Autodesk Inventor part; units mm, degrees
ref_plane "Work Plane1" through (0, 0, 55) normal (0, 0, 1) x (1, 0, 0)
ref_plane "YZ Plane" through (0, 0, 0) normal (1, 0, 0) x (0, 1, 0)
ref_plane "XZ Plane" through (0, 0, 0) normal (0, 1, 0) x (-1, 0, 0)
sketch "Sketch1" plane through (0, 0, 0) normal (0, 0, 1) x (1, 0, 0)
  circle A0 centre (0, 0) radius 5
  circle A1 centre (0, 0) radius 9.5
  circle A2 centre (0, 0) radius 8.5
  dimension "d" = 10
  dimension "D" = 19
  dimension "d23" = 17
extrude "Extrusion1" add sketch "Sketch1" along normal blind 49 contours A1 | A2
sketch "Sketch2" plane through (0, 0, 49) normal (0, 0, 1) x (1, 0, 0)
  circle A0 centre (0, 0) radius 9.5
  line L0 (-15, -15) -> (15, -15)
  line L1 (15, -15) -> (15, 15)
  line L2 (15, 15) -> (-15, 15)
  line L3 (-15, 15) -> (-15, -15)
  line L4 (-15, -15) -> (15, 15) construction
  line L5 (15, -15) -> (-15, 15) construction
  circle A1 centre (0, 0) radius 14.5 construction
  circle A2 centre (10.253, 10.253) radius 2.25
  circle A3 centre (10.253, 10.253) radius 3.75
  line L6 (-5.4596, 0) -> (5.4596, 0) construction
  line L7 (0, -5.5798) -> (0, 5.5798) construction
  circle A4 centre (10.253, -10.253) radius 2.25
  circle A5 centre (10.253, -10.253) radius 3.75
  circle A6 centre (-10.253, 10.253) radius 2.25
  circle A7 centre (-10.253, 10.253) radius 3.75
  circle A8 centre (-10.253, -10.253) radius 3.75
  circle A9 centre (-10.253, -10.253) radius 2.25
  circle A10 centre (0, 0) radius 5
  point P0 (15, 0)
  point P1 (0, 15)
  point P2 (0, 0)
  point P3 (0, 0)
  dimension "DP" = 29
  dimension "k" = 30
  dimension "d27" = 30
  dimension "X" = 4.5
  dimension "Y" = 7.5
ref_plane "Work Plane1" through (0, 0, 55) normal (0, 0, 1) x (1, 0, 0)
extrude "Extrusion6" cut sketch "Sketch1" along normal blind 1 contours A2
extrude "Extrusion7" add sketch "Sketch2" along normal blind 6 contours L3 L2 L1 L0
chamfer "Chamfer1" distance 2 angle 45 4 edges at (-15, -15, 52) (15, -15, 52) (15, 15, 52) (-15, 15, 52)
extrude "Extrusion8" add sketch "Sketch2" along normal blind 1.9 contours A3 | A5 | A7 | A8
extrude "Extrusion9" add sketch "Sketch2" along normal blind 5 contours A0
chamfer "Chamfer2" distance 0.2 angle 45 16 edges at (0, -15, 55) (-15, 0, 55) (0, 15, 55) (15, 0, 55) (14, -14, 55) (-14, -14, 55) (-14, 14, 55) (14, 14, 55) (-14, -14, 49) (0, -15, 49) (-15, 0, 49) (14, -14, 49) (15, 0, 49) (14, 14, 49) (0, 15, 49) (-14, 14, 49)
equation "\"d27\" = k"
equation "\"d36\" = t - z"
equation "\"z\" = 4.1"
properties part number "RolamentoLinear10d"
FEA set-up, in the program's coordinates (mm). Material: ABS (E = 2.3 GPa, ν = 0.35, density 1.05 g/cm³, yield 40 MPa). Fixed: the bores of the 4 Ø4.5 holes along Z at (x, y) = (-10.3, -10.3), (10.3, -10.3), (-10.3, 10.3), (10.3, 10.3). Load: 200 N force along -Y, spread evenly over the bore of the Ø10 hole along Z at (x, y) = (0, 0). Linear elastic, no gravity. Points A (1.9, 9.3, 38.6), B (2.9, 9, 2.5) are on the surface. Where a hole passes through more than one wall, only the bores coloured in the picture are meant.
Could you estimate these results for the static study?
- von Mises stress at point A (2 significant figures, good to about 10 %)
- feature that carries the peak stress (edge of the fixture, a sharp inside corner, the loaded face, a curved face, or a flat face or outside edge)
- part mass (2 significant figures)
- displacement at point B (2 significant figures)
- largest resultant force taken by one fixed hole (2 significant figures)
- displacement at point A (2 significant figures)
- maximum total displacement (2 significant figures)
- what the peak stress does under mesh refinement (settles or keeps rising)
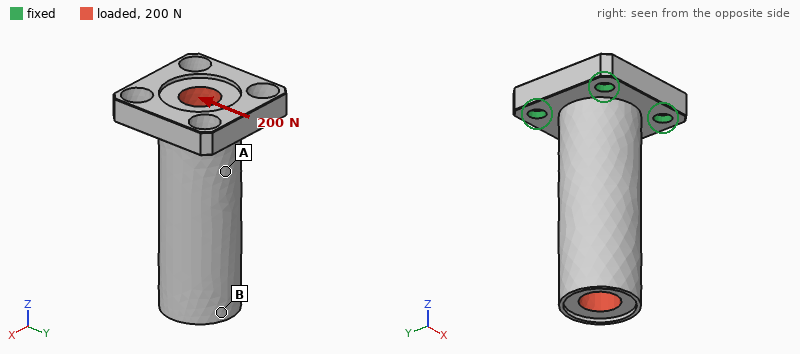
4.0 MPa
edge of the fixture
14 g
0.47 mm
130 N
0.12 mm
0.49 mm
keeps rising
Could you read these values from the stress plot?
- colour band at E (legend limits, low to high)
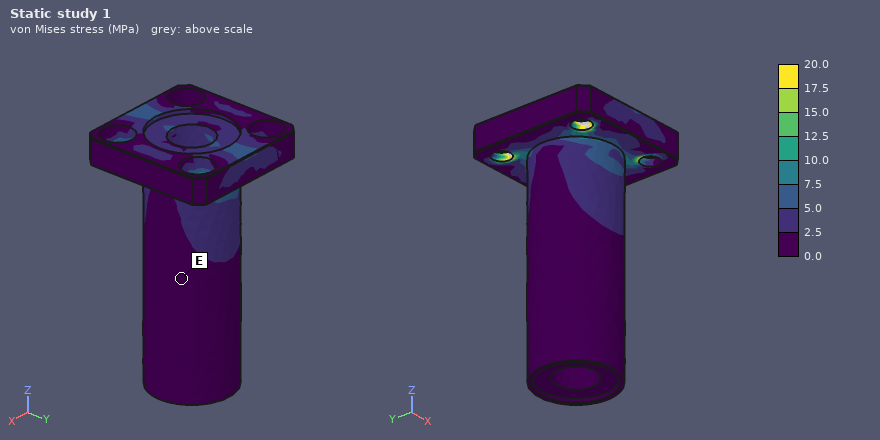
0.0 to 2.5 MPa
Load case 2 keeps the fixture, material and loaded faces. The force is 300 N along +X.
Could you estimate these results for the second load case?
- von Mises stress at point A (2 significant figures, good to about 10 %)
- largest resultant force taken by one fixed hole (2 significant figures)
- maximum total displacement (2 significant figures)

2.7 MPa
190 N
0.74 mm
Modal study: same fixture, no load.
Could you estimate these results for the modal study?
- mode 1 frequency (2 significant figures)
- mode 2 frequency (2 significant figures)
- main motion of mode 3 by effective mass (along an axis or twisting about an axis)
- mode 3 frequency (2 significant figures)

1200 Hz
1200 Hz
along Z
4200 Hz
